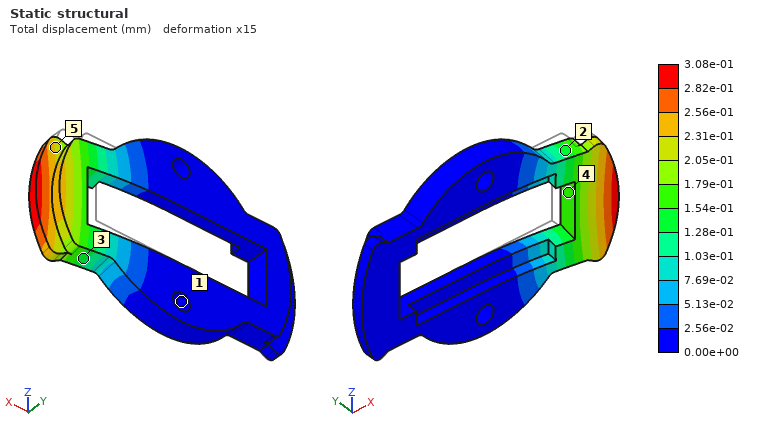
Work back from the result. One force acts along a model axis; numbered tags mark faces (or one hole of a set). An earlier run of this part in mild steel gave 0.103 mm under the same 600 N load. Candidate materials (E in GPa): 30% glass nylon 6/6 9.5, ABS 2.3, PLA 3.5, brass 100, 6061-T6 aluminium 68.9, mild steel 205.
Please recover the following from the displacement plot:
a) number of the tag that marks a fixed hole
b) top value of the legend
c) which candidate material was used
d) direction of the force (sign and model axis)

1
3.08e-01 mm
6061-T6 aluminium
-Y
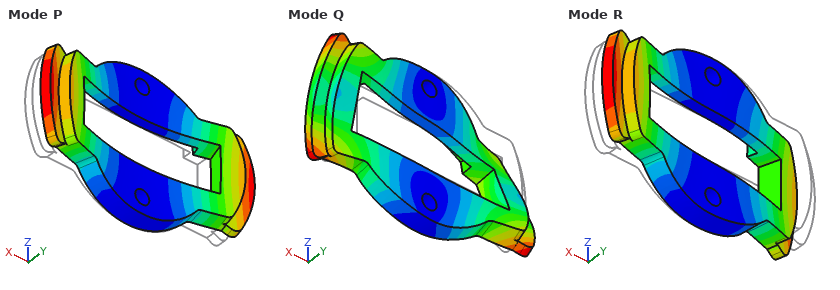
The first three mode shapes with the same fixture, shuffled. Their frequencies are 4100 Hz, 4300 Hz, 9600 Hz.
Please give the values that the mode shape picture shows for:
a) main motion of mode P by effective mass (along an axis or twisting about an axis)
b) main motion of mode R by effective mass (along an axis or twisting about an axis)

along Y
twisting about Z
